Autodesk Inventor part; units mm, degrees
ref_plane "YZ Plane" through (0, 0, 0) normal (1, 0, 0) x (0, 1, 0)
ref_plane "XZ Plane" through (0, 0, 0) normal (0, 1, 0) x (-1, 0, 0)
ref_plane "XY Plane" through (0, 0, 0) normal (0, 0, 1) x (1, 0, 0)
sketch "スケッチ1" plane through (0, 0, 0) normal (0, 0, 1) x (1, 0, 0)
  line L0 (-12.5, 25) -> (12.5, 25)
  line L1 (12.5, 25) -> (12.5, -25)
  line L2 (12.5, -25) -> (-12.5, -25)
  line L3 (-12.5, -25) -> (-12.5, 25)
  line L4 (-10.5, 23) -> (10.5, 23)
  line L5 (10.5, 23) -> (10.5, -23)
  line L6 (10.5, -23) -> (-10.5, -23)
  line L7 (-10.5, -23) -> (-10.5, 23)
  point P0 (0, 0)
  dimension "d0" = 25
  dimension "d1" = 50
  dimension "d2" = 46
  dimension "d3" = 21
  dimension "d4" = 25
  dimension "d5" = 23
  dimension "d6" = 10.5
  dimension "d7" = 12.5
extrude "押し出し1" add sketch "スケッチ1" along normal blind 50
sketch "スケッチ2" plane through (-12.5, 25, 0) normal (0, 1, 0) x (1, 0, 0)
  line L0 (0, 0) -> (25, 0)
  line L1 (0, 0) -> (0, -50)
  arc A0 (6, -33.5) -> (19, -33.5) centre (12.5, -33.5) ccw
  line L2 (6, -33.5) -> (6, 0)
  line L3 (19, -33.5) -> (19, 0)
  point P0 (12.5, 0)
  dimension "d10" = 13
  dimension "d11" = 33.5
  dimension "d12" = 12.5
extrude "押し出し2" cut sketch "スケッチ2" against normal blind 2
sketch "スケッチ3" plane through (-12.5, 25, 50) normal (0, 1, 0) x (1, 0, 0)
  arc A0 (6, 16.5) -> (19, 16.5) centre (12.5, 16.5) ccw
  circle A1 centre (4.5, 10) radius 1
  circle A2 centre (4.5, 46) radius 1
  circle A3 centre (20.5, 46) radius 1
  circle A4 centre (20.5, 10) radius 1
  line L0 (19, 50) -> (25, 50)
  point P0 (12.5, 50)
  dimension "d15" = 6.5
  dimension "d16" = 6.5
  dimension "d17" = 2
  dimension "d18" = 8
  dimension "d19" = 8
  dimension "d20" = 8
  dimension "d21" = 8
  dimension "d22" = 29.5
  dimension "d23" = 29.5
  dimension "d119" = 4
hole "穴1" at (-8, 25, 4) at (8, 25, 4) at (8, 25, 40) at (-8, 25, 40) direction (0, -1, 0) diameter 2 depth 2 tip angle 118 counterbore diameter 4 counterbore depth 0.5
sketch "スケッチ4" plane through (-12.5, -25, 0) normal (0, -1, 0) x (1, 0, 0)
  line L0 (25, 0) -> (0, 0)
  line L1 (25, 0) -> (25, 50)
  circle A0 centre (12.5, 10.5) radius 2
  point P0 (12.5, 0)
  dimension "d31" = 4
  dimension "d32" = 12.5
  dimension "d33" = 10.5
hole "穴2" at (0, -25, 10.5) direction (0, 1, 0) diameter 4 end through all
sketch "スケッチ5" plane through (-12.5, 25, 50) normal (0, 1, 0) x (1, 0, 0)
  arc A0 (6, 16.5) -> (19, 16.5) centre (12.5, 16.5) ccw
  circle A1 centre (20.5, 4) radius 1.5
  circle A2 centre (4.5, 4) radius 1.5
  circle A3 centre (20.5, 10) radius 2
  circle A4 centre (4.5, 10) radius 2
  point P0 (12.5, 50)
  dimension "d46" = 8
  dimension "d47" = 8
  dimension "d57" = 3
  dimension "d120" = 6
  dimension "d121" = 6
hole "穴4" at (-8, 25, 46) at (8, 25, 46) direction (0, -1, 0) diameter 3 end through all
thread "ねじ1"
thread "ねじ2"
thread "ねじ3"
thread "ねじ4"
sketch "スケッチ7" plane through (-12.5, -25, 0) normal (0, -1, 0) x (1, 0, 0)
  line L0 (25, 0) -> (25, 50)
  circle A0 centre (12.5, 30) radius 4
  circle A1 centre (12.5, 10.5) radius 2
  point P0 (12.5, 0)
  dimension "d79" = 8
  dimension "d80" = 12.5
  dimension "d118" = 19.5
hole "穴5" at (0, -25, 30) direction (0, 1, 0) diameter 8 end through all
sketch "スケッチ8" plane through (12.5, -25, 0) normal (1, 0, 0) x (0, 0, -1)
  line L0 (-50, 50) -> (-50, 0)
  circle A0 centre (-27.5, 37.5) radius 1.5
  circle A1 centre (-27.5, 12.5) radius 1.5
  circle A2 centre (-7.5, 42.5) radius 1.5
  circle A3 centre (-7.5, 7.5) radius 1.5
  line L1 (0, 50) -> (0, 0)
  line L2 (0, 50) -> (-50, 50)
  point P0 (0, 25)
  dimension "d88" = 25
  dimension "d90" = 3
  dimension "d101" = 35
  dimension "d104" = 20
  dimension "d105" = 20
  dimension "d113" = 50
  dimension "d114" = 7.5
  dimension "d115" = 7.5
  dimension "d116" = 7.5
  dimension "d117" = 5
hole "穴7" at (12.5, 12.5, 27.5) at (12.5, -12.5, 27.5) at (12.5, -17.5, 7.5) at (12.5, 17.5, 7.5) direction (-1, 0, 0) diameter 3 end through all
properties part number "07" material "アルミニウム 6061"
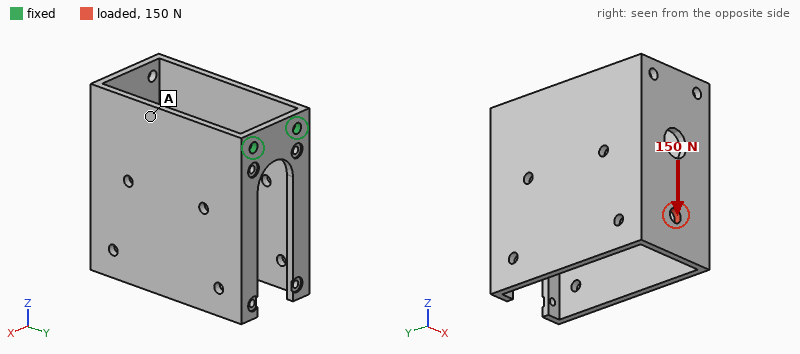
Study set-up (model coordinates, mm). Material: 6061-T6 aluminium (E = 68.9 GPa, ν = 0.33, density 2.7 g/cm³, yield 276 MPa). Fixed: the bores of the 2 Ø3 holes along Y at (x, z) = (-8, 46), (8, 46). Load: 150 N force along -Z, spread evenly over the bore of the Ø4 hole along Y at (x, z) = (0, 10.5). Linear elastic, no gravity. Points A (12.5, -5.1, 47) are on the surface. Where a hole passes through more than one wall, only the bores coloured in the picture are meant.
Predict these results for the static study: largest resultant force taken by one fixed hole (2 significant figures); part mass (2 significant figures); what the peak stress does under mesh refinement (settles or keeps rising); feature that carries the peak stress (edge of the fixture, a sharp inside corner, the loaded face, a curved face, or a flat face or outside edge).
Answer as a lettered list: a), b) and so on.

a) 76 N
b) 35 g
c) keeps rising
d) edge of the fixture
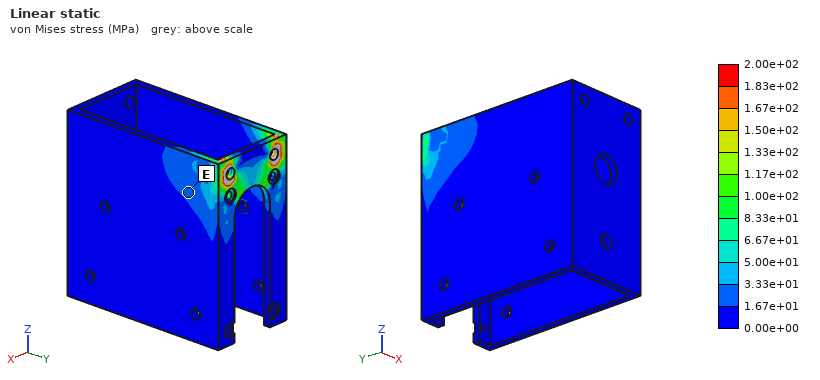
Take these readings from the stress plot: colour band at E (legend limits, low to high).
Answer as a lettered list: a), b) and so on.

a) 1.67e+01 to 3.33e+01 MPa
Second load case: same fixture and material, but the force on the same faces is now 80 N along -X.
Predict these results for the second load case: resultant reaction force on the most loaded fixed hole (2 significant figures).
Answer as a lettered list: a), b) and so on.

a) 190 N
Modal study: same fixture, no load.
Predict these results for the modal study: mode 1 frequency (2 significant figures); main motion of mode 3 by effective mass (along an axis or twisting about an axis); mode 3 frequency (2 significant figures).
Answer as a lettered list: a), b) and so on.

a) 560 Hz
b) twisting about Y
c) 1100 Hz
